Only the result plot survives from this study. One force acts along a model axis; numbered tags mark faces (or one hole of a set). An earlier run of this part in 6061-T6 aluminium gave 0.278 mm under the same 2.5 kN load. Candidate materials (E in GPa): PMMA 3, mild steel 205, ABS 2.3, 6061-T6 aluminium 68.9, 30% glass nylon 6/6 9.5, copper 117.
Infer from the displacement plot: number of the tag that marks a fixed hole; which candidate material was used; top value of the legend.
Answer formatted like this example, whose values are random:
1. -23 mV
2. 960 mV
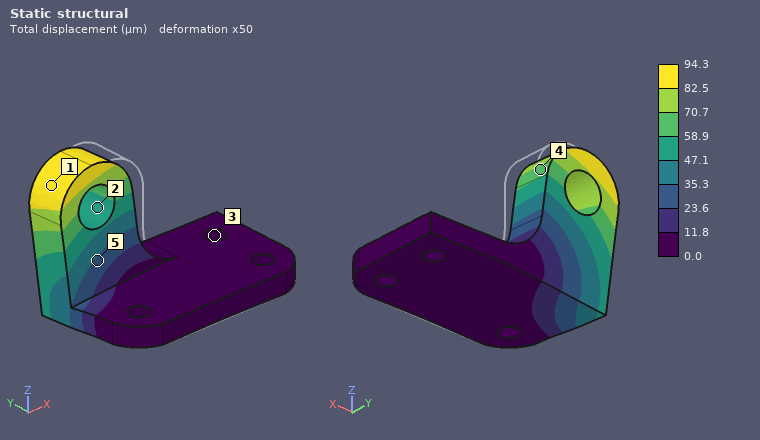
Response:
1. 3
2. mild steel
3. 94.3 µm
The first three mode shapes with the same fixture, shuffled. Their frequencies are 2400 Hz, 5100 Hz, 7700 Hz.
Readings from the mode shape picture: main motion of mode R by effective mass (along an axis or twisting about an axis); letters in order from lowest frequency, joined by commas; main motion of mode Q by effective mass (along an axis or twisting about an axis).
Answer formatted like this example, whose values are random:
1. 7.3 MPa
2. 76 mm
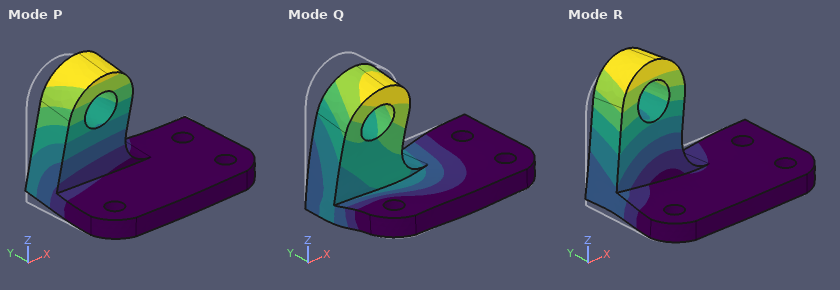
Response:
1. along X
2. P, R, Q
3. along Z
